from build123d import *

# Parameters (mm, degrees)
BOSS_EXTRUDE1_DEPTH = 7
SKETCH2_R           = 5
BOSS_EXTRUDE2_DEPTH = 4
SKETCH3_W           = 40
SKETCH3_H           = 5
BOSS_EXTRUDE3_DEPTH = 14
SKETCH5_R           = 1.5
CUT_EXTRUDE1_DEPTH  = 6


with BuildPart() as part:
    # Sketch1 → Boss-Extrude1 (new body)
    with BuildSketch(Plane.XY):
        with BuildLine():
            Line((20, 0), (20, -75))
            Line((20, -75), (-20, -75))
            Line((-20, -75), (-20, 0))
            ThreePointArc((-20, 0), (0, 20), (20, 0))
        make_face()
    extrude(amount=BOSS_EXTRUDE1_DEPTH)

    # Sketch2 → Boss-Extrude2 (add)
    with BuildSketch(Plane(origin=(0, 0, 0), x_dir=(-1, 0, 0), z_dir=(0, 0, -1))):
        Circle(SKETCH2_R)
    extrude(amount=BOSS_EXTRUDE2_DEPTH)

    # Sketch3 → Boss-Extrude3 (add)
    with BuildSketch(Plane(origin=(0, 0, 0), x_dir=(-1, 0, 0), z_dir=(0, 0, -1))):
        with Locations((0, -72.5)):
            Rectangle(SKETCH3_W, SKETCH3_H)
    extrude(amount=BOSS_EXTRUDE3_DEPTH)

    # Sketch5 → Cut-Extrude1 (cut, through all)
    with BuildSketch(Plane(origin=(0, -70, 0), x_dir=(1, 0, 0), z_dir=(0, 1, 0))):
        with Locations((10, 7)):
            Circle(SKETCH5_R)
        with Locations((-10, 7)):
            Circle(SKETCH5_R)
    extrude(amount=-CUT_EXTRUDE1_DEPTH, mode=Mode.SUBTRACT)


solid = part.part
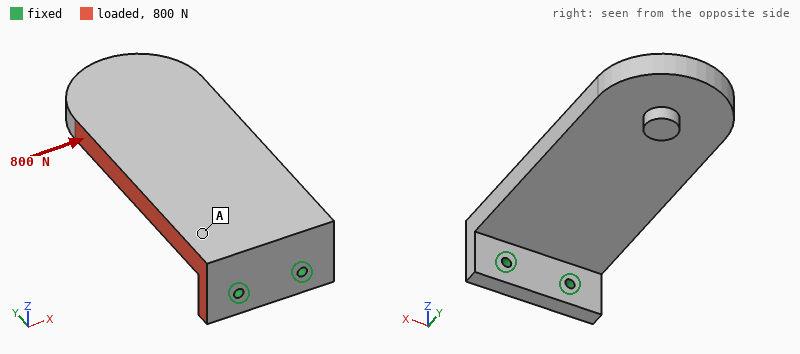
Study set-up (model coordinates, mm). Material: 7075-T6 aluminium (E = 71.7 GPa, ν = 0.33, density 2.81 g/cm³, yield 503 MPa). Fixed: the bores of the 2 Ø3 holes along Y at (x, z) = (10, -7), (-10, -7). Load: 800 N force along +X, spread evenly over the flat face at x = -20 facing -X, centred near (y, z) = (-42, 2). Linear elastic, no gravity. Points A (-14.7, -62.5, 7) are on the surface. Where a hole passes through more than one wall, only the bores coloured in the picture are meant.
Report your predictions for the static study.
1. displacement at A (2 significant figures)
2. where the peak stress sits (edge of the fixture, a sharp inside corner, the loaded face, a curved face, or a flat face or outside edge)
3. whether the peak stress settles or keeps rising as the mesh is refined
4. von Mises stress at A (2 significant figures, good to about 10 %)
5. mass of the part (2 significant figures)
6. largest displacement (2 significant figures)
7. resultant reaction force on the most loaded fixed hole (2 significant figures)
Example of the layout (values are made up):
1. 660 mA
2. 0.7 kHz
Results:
1. 0.030 mm
2. edge of the fixture
3. keeps rising
4. 11 MPa
5. 80 g
6. 0.16 mm
7. 1.2 kN
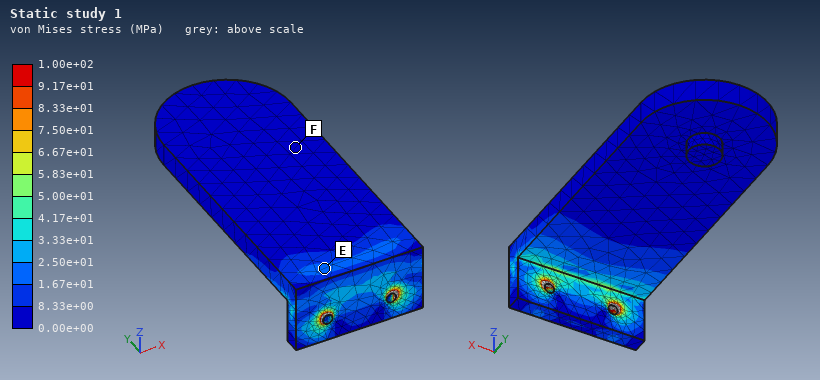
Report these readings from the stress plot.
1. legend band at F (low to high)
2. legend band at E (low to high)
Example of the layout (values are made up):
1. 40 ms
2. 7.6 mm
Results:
1. 0.00e+00 to 8.33e+00 MPa
2. 1.67e+01 to 2.50e+01 MPa
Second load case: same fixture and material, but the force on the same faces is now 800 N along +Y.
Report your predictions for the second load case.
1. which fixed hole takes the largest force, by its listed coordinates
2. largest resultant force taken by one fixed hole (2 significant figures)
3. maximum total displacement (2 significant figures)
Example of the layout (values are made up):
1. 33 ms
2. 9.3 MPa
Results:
1. (-10, -7)
2. 1.0 kN
3. 0.18 mm
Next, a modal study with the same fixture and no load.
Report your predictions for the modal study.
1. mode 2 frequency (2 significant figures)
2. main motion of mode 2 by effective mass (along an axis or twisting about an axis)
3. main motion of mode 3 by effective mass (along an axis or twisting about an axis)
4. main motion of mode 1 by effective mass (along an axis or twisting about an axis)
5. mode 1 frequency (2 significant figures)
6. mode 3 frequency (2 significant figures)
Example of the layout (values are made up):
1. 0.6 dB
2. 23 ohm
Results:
1. 1400 Hz
2. along X
3. twisting about Y
4. along Z
5. 480 Hz
6. 3200 Hz
